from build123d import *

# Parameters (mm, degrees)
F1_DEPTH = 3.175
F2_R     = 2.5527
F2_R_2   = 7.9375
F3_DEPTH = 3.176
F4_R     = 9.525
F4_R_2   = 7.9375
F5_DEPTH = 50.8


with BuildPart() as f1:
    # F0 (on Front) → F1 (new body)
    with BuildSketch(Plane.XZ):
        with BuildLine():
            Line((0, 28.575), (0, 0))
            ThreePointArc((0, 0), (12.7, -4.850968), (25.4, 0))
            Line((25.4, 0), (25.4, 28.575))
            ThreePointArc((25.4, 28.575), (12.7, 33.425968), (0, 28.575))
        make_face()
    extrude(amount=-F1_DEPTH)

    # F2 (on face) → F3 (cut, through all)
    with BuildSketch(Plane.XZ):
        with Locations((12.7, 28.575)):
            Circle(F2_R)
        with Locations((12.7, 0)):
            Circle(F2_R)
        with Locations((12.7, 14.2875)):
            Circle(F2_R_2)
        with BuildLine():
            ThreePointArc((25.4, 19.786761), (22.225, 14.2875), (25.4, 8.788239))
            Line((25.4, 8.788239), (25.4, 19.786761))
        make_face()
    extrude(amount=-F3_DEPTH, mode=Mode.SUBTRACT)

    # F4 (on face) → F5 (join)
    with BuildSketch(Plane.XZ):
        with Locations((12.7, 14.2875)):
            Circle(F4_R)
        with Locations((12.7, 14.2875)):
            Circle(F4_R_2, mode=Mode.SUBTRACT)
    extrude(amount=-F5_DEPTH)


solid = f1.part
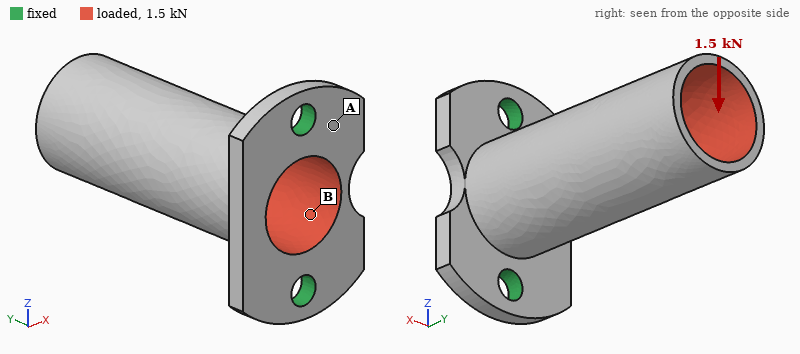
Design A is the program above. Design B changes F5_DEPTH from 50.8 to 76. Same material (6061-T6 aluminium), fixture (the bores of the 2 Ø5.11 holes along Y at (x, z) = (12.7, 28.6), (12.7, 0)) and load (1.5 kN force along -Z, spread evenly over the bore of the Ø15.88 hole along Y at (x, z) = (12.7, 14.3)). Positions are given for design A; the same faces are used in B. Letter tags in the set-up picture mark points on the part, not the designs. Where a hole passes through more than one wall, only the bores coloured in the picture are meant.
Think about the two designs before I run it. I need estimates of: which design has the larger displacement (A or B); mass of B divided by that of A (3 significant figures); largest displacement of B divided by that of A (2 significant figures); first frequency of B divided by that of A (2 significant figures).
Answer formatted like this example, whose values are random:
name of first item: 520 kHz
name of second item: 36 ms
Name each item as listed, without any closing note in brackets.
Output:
which design has the larger displacement: B
mass of B divided by that of A: 1.36
largest displacement of B divided by that of A: 2.7
first frequency of B divided by that of A: 0.54
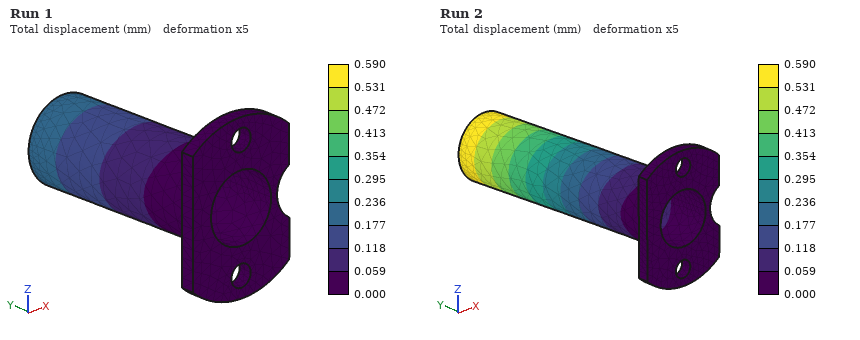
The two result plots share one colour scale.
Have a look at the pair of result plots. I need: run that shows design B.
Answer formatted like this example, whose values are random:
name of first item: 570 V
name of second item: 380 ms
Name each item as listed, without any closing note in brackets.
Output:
run that shows design B: Run 2
